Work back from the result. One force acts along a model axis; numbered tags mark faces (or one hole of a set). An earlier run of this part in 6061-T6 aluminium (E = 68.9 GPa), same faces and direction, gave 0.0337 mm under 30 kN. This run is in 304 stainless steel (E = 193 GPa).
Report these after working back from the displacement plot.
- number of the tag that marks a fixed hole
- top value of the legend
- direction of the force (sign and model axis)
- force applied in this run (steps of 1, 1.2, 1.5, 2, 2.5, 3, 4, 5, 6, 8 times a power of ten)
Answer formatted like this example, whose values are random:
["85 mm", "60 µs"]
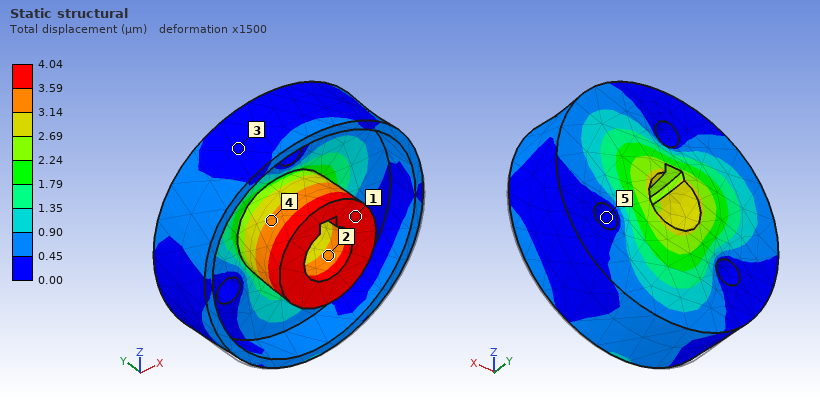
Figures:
["5", "4.04 µm", "+Y", "10 kN"]
